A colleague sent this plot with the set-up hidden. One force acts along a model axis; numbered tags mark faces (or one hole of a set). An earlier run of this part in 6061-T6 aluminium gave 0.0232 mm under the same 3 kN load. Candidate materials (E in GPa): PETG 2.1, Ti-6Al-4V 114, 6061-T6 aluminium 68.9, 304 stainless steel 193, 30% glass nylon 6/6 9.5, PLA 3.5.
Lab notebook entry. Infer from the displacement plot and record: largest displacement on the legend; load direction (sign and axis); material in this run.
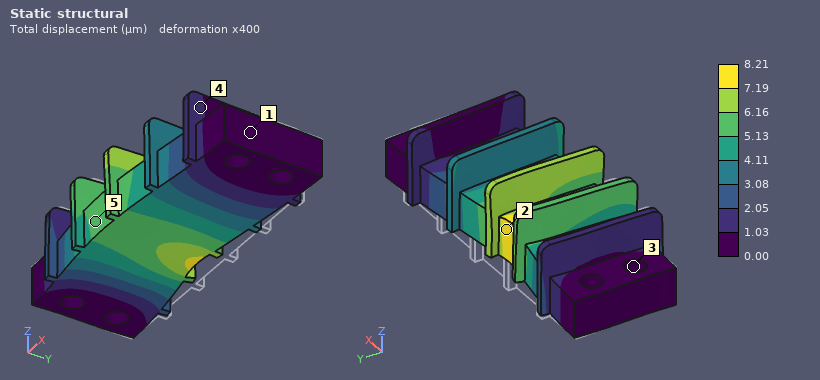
8.21 µm
-Y
304 stainless steel
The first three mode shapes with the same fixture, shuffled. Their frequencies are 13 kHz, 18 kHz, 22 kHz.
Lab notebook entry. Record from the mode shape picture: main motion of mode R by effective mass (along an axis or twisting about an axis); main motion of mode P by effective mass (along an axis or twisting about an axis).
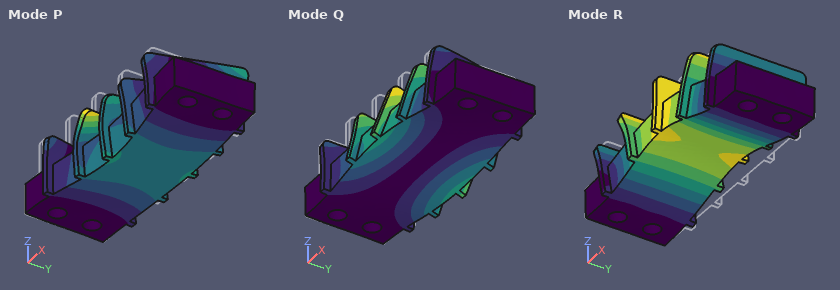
along Z
along Y
